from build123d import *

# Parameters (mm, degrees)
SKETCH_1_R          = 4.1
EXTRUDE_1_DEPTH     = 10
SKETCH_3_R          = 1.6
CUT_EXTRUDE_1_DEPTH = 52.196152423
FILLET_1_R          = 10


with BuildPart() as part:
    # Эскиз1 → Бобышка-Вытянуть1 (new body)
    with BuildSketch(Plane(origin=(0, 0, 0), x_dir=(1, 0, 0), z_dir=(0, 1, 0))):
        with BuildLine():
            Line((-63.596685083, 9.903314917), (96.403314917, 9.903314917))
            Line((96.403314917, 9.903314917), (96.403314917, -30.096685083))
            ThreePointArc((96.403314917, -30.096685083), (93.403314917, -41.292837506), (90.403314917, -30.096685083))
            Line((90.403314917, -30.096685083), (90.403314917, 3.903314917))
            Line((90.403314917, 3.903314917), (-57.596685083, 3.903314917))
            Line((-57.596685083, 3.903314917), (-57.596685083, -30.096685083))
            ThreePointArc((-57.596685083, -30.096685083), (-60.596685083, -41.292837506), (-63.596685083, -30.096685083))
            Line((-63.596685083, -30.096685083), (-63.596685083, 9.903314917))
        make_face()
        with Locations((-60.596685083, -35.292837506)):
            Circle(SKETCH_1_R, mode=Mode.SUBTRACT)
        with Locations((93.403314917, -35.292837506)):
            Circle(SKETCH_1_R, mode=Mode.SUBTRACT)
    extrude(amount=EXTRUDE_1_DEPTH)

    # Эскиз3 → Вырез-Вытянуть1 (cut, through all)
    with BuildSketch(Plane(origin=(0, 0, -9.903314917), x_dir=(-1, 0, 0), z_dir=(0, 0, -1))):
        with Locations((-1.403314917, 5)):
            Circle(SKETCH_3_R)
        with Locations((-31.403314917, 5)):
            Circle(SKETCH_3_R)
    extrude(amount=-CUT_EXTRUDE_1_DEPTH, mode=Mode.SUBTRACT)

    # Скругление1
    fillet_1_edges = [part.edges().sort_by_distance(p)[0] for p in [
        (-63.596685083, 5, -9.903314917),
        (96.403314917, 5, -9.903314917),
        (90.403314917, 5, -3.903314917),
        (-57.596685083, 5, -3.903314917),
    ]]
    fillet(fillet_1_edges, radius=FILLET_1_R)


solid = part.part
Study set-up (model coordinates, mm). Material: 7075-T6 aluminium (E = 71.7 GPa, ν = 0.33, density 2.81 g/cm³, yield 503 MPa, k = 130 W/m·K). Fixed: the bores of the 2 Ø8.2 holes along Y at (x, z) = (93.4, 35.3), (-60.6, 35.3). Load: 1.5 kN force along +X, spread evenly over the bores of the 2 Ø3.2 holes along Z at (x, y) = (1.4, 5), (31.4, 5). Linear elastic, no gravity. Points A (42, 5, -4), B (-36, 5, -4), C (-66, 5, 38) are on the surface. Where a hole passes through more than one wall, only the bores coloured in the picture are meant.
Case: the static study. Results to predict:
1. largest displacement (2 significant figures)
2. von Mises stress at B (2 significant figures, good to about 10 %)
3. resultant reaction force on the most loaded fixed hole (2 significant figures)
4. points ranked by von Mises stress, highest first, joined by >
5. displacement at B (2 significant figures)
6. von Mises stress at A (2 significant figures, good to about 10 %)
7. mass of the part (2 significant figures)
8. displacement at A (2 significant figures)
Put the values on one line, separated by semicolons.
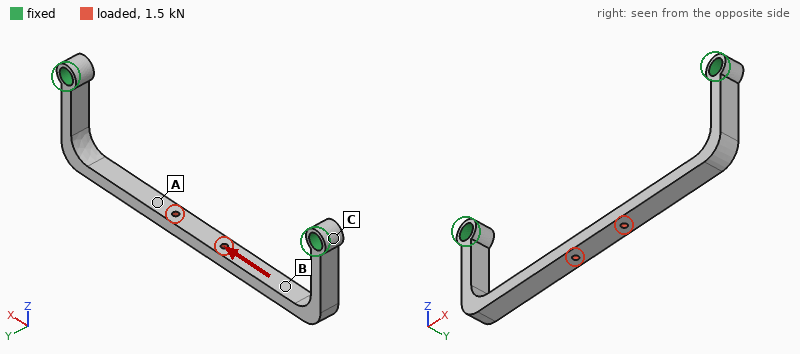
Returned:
0.60 mm; 130 MPa; 760 N; B > A > C; 0.58 mm; 69 MPa; 41 g; 0.59 mm
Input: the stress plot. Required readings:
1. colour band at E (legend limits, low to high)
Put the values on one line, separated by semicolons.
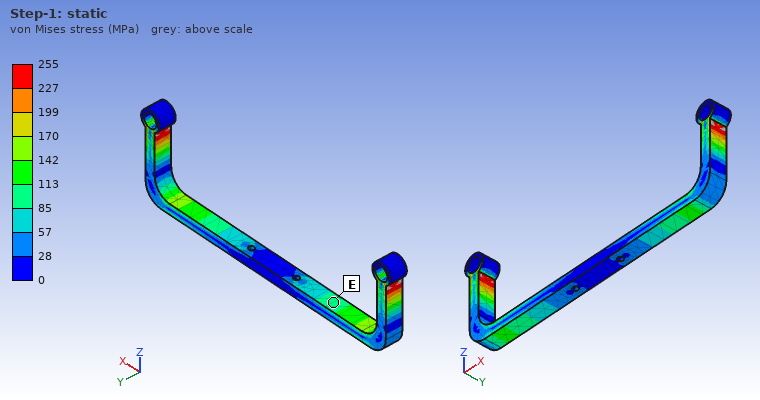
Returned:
85 to 113 MPa
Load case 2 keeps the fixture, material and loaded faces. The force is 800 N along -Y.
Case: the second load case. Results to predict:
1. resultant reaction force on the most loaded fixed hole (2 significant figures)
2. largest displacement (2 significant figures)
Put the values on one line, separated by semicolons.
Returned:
400 N; 1.3 mm
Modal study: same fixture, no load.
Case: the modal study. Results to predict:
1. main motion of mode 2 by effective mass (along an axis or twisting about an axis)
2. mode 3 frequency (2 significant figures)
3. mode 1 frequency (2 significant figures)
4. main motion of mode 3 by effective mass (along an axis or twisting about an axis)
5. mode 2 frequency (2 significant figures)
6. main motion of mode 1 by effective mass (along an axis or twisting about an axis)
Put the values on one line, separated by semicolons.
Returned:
along Z; 1500 Hz; 1100 Hz; along X; 1300 Hz; along Y
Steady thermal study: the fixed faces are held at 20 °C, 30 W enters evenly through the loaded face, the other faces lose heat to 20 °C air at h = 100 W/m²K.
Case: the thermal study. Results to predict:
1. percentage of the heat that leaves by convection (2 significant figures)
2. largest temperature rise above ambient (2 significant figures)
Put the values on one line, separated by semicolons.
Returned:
77 %; 73 K
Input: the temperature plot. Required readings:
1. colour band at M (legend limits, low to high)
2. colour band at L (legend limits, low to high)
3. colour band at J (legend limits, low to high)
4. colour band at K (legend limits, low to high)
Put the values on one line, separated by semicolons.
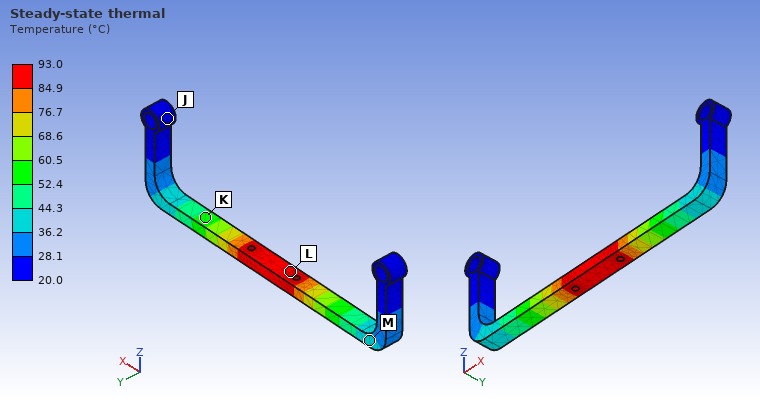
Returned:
36.2 to 44.3 °C; 84.9 to 93.0 °C; 20.0 to 28.1 °C; 52.4 to 60.5 °C
